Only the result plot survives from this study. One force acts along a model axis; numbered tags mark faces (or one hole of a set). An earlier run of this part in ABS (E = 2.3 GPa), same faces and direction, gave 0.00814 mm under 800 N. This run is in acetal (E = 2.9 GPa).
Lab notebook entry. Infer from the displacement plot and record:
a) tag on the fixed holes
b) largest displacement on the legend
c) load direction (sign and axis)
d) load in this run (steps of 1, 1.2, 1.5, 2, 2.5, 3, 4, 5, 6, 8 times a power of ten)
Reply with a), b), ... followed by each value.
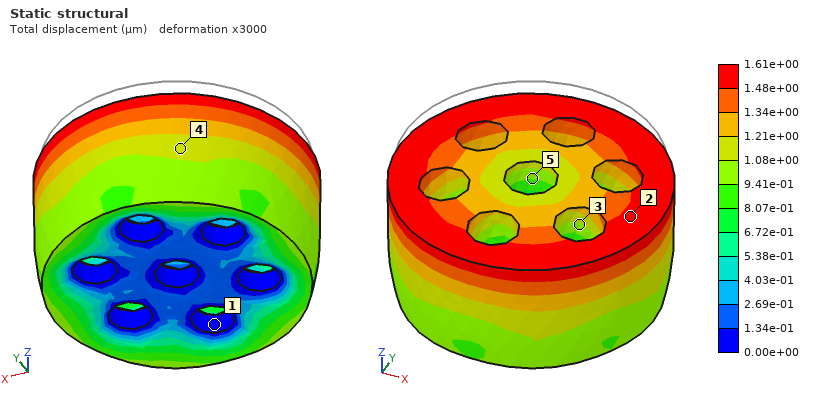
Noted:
a) 1
b) 1.61e+00 µm
c) -Z
d) 200 N
